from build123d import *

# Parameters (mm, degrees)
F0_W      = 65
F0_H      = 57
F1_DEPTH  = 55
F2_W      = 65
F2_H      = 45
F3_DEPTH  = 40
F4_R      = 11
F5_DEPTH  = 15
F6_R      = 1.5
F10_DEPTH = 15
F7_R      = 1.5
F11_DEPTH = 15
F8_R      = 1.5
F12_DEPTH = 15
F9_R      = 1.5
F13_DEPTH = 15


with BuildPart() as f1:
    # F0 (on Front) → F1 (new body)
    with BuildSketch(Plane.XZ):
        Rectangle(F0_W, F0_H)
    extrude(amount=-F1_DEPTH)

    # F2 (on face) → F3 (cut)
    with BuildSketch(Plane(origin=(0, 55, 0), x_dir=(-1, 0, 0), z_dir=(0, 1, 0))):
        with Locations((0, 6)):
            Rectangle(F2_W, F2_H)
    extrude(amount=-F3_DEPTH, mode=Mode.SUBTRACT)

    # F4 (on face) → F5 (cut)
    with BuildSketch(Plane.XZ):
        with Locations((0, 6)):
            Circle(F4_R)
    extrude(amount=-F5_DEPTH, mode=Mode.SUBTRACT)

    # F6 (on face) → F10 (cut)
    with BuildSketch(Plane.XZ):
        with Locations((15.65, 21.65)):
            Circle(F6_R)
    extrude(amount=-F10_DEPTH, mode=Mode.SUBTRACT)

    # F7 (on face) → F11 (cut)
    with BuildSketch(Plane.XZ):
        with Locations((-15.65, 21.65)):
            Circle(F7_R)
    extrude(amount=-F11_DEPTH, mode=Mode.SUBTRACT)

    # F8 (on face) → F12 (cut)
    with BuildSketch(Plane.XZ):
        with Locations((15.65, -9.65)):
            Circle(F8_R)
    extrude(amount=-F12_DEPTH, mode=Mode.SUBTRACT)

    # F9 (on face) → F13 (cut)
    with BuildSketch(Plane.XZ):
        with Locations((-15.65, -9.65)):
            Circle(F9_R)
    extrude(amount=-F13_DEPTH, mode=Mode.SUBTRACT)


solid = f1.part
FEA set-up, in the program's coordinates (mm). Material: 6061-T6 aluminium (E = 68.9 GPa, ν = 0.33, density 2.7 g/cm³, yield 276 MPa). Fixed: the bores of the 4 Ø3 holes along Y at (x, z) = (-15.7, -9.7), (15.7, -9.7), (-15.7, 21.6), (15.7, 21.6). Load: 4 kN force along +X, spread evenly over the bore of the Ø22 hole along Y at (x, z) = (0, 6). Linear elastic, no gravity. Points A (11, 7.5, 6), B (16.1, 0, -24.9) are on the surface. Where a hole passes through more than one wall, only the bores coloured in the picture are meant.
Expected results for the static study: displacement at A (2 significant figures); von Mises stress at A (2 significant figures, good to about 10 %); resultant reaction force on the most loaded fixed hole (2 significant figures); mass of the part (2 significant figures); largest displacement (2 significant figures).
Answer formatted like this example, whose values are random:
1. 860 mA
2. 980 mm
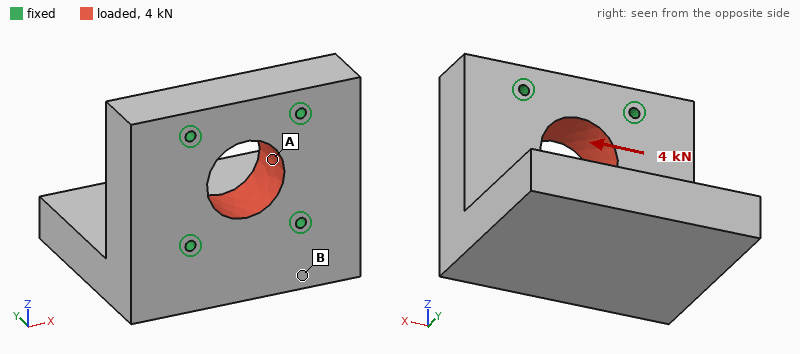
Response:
1. 1.5 µm
2. 3.7 MPa
3. 1.0 kN
4. 220 g
5. 1.6 µm
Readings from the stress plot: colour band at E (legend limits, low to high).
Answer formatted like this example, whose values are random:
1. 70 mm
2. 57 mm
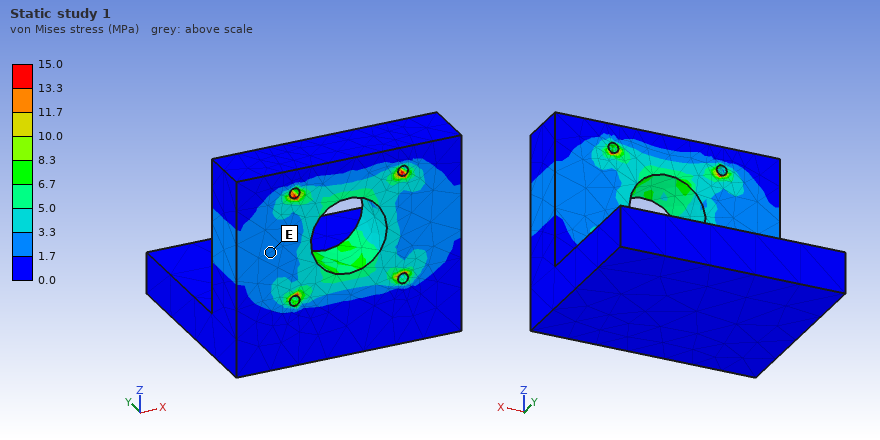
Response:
1. 1.7 to 3.3 MPa
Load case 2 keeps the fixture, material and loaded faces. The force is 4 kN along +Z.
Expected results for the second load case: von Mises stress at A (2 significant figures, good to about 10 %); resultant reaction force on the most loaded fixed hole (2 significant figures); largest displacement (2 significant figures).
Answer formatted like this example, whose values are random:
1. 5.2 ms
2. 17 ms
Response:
1. 6.7 MPa
2. 1.0 kN
3. 2.3 µm
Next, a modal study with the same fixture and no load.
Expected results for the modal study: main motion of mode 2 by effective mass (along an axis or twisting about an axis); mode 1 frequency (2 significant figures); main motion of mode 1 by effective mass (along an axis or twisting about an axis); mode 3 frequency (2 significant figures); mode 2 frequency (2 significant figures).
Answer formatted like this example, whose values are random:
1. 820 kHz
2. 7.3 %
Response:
1. along X
2. 3400 Hz
3. along Z
4. 7800 Hz
5. 6100 Hz
